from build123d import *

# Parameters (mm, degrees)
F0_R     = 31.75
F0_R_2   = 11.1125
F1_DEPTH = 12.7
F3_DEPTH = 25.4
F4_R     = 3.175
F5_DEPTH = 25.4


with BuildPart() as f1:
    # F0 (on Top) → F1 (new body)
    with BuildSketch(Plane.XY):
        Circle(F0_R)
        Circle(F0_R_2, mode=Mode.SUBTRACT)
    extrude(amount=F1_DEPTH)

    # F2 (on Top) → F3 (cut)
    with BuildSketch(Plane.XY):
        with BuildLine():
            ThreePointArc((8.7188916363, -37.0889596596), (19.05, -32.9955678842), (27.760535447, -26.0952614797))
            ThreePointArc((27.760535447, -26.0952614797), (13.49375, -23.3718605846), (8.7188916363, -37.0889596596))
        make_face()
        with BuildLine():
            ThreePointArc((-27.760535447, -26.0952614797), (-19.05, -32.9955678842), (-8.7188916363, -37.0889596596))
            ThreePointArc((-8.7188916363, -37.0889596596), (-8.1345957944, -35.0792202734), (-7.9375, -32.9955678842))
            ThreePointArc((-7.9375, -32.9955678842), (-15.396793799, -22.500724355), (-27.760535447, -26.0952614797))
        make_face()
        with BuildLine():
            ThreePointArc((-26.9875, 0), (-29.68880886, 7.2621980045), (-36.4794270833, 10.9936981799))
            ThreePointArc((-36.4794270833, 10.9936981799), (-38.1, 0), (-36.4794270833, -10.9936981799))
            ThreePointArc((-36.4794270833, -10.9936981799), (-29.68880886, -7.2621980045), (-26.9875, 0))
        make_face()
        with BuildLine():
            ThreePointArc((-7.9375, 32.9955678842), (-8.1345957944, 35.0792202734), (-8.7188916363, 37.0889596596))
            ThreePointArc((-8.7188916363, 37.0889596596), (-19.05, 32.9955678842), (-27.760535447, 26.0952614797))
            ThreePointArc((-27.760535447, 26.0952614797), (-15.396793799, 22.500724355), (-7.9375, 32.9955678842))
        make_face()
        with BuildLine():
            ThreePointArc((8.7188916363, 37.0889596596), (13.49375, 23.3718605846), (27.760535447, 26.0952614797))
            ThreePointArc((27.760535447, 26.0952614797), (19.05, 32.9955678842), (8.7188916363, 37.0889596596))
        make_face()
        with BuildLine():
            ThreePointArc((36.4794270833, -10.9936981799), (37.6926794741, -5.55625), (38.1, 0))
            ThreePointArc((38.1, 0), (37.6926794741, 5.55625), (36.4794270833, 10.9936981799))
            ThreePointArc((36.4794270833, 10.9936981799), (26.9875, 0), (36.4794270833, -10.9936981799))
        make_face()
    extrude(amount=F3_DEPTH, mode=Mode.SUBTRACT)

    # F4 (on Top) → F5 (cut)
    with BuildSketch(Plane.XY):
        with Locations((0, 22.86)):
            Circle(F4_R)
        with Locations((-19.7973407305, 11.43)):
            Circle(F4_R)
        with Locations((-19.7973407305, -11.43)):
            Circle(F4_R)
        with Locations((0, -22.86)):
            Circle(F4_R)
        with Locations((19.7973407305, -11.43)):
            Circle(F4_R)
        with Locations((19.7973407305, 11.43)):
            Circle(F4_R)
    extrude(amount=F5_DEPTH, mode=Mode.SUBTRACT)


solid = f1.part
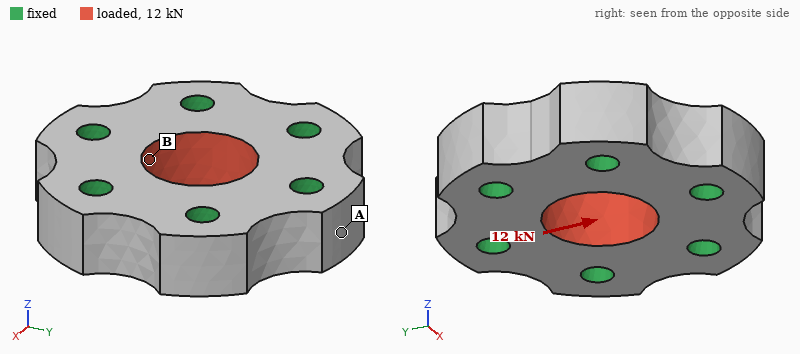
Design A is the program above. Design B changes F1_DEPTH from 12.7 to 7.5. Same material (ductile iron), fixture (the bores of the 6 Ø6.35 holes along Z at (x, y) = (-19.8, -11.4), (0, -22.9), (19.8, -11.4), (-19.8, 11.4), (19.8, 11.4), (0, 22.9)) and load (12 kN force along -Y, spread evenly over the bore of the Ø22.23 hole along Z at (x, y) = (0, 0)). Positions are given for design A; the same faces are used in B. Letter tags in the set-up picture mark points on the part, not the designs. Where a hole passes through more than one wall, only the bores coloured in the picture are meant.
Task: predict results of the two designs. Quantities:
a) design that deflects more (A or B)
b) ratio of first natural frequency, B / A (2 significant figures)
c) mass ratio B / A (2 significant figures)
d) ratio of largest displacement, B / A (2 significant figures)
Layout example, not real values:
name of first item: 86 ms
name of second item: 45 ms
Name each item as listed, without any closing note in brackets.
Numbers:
design that deflects more: B
ratio of first natural frequency, B / A: 0.83
mass ratio B / A: 0.59
ratio of largest displacement, B / A: 1.7
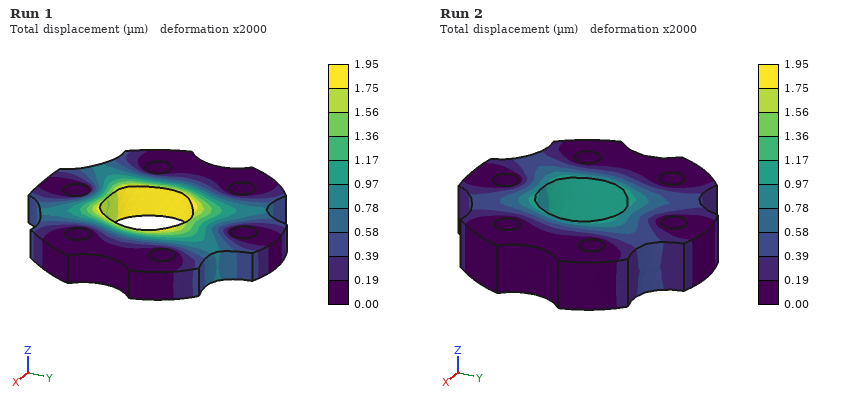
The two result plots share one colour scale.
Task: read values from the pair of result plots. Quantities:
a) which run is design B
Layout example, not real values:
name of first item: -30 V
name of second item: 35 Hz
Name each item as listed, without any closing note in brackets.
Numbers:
which run is design B: Run 1
